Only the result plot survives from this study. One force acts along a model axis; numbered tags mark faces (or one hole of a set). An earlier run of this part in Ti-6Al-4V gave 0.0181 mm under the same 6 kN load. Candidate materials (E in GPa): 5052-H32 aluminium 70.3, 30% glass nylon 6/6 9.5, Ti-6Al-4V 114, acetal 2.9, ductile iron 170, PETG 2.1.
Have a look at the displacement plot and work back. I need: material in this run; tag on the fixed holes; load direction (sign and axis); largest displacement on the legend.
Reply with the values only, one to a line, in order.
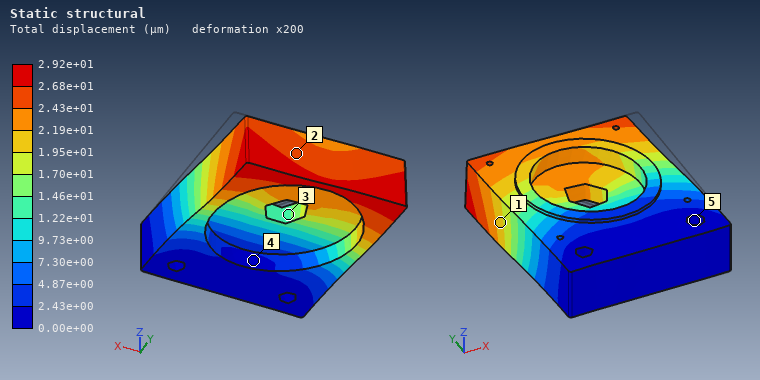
5052-H32 aluminium
5
-X
2.92e+01 µm
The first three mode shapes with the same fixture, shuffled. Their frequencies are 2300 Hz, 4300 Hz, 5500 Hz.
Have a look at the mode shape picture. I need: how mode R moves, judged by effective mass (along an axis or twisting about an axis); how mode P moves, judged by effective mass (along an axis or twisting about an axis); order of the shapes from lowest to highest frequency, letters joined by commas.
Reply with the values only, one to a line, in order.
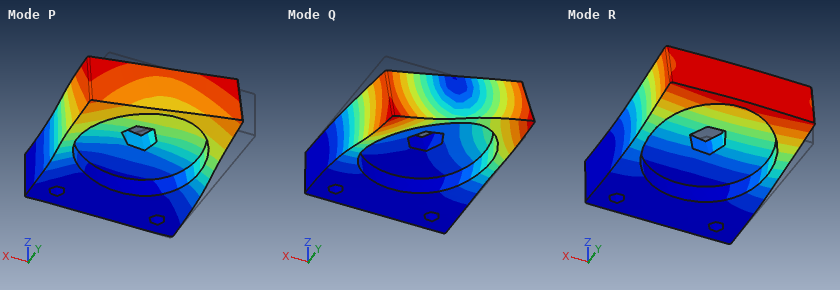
along Z
along X
R, Q, P
